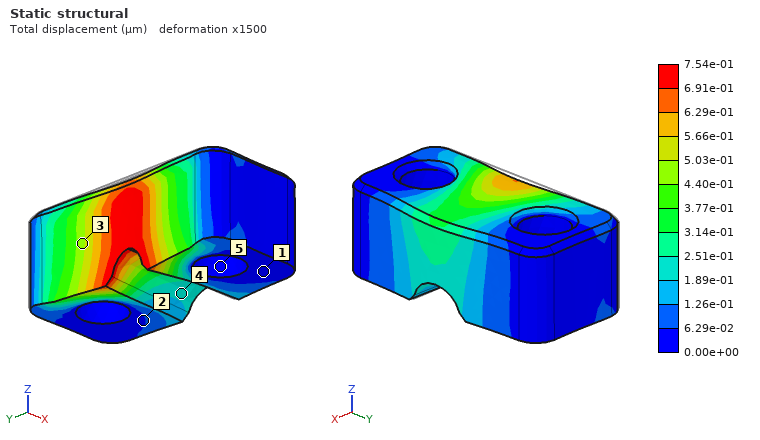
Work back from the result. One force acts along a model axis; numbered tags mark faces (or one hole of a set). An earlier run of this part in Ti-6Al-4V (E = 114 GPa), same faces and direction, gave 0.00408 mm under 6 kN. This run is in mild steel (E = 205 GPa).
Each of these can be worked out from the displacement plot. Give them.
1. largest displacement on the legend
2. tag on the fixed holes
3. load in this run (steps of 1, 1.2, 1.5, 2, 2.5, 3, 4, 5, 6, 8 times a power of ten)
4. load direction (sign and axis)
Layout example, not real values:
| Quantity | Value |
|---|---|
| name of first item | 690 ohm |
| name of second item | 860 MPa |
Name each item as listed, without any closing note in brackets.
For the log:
| Quantity | Value |
|---|---|
| largest displacement on the legend | 7.54e-01 µm |
| tag on the fixed holes | 5 |
| load in this run | 2 kN |
| load direction | +X |
